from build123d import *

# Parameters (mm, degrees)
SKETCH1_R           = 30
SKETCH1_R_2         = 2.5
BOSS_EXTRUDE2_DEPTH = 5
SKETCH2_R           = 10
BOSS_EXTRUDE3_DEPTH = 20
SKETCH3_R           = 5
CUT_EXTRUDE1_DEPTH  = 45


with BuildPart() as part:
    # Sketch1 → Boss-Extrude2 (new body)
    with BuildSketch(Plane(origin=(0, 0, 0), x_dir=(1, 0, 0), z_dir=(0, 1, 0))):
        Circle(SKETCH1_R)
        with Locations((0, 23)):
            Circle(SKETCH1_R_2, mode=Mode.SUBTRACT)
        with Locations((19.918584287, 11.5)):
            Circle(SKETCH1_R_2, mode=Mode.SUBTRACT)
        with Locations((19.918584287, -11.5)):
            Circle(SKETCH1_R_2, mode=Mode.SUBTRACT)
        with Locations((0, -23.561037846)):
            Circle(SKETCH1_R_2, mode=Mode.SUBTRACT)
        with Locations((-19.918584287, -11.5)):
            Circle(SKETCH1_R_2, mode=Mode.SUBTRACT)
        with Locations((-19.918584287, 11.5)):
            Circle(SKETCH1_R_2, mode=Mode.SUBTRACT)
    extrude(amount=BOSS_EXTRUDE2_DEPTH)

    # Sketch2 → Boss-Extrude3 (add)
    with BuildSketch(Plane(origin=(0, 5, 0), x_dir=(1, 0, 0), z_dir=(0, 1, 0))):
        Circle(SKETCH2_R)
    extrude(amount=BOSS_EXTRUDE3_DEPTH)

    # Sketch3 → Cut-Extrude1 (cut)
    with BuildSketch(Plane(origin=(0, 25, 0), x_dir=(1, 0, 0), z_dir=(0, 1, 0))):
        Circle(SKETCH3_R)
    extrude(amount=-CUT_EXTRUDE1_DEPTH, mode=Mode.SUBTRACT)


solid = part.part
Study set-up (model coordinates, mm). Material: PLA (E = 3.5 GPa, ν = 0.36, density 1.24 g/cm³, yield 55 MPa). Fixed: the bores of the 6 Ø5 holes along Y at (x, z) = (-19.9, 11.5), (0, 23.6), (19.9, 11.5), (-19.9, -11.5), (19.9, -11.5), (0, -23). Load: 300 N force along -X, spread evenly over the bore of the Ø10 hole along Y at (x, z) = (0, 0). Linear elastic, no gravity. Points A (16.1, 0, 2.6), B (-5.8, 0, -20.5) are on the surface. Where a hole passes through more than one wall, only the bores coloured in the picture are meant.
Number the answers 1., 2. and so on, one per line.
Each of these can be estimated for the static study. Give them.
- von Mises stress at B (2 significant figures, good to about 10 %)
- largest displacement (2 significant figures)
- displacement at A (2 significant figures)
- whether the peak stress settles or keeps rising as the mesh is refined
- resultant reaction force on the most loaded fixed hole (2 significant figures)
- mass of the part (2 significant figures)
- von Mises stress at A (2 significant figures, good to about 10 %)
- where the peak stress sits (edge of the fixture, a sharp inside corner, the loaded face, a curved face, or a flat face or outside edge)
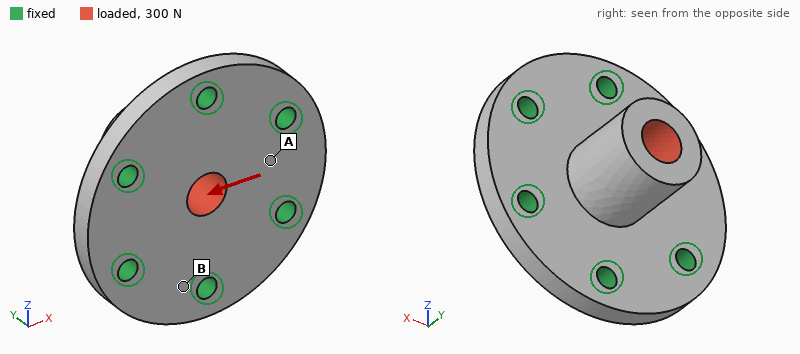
1. 0.80 MPa
2. 79 µm
3. 12 µm
4. keeps rising
5. 86 N
6. 22 g
7. 1.6 MPa
8. edge of the fixture
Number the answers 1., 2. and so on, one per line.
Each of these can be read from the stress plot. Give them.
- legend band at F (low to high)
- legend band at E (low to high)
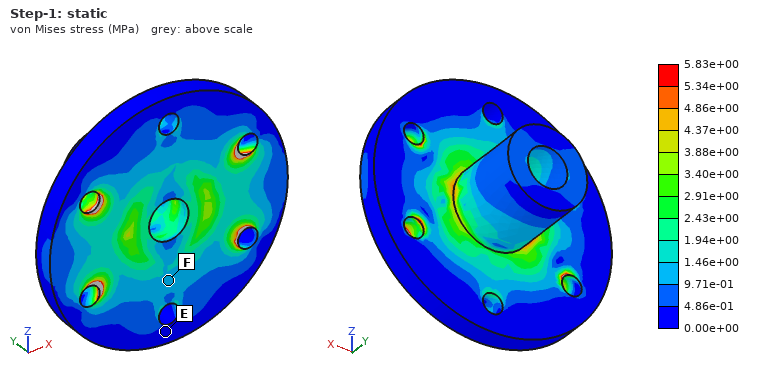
1. 9.71e-01 to 1.46e+00 MPa
2. 0.00e+00 to 4.86e-01 MPa
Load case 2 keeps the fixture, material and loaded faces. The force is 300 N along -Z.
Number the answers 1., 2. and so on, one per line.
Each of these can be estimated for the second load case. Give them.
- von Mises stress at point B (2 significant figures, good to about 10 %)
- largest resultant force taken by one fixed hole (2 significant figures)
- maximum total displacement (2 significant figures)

1. 1.6 MPa
2. 99 N
3. 80 µm
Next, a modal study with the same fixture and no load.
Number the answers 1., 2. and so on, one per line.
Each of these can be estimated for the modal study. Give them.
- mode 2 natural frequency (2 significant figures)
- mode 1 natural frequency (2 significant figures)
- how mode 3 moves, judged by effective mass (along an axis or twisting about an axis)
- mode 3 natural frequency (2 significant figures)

1. 4200 Hz
2. 4100 Hz
3. along Y
4. 5000 Hz
